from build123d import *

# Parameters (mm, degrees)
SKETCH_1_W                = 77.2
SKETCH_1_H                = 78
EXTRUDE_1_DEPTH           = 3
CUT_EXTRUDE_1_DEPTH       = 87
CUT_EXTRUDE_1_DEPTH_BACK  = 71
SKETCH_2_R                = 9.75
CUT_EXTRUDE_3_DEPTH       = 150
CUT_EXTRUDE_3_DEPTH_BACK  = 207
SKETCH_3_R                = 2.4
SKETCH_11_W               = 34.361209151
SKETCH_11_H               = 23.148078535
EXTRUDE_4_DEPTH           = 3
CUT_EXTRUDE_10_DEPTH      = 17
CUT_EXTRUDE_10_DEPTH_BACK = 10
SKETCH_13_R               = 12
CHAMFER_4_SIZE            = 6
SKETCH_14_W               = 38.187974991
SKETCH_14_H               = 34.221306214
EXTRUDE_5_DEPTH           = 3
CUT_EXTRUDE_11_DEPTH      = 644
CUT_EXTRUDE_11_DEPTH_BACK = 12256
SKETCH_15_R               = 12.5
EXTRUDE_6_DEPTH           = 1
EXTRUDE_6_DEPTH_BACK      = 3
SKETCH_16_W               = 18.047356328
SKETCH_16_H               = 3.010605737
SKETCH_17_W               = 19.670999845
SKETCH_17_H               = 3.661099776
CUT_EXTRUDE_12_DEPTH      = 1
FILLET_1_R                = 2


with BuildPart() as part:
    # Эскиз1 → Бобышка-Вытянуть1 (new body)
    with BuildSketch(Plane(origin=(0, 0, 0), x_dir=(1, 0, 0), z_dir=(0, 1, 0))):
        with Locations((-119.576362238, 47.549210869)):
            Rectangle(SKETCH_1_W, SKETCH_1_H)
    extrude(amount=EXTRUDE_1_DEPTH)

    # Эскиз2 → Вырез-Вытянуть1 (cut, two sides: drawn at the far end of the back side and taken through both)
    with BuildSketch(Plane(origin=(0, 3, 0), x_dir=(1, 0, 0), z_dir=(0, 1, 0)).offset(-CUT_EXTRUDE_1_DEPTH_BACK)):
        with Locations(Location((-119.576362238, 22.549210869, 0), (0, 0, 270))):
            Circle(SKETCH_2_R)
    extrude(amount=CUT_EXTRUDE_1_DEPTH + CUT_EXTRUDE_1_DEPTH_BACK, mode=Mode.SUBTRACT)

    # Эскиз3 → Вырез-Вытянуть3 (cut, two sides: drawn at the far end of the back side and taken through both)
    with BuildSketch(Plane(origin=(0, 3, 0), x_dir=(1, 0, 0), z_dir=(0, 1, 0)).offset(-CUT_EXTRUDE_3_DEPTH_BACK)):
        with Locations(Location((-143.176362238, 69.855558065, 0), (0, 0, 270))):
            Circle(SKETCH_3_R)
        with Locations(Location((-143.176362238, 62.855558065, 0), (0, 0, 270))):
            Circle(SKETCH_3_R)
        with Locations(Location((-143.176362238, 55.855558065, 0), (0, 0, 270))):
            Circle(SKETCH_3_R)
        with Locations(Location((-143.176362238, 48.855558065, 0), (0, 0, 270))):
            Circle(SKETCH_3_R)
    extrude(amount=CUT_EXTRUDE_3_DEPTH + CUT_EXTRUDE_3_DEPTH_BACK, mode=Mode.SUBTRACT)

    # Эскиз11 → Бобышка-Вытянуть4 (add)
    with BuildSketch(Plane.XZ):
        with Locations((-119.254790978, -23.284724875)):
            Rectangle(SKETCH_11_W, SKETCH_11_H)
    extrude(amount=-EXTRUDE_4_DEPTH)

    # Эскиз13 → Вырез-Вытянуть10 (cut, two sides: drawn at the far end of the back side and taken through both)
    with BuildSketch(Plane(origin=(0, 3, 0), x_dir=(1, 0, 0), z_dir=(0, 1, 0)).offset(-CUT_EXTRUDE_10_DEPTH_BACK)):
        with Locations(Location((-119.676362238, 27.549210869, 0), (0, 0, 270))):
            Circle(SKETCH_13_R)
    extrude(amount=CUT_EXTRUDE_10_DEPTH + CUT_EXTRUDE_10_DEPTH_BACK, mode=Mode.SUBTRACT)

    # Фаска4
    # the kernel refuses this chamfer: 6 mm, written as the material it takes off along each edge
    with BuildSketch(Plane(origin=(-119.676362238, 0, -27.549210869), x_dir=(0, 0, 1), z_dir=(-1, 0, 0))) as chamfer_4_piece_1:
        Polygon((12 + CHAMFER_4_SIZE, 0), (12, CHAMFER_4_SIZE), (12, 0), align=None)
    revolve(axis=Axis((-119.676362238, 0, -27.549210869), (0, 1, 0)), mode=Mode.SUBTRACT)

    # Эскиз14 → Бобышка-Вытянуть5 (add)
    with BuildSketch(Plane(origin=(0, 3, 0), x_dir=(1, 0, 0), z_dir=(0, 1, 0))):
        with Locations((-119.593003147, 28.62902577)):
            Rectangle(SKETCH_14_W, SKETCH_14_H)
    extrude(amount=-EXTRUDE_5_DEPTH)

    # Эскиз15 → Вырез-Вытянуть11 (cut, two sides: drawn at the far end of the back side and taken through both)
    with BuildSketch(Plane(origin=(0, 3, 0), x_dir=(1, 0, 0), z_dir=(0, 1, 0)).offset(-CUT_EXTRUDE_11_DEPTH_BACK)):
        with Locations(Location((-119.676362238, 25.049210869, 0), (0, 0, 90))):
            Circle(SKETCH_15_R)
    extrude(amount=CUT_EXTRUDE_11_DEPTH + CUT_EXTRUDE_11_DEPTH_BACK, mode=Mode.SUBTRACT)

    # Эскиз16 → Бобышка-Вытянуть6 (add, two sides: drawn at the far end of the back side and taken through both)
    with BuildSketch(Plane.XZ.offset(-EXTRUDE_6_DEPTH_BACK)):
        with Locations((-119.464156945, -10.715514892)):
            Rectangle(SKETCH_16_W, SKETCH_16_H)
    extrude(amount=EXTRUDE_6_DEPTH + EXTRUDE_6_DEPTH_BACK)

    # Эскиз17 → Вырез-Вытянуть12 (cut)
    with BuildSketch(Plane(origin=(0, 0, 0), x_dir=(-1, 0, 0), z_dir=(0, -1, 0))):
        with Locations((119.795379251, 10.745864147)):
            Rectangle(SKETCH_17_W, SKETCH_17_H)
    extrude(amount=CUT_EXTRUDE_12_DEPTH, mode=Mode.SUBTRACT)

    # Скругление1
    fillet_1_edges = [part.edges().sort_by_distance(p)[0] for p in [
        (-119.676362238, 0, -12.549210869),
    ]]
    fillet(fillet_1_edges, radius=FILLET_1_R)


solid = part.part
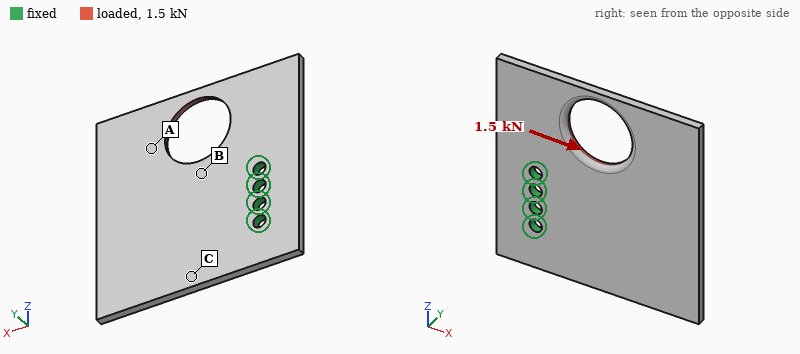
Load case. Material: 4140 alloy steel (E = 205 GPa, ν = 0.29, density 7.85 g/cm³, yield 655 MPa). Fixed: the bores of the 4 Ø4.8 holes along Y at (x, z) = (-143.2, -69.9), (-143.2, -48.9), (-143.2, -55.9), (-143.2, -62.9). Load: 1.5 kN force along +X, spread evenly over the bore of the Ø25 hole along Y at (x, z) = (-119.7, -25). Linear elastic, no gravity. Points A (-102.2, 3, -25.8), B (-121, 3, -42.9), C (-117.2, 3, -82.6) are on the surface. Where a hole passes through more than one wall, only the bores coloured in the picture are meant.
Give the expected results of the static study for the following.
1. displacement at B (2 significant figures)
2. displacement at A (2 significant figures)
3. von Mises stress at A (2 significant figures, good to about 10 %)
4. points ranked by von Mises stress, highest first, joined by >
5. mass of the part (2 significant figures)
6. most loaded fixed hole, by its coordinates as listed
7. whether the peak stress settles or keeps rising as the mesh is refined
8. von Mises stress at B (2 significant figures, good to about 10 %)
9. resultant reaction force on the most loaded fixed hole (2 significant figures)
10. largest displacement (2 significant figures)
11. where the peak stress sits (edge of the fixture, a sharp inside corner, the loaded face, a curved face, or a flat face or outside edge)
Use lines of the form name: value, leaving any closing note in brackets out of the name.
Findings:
displacement at B: 0.016 mm
displacement at A: 0.052 mm
von Mises stress at A: 21 MPa
points ranked by von Mises stress, highest first, joined by >: B > A > C
mass of the part: 130 g
most loaded fixed hole, by its coordinates as listed: (-143.2, -48.9)
whether the peak stress settles or keeps rising as the mesh is refined: keeps rising
von Mises stress at B: 37 MPa
resultant reaction force on the most loaded fixed hole: 2.5 kN
largest displacement: 0.10 mm
where the peak stress sits: edge of the fixture
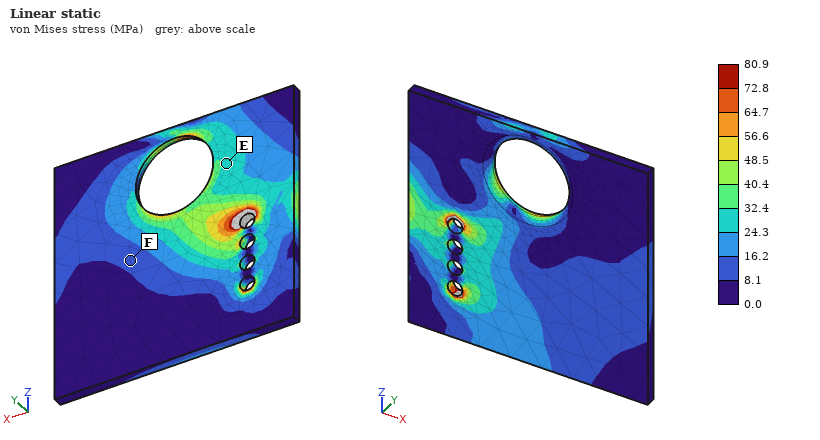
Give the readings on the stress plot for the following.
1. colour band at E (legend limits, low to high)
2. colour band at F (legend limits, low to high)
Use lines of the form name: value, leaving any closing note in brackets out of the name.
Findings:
colour band at E: 24.3 to 32.4 MPa
colour band at F: 8.1 to 16.2 MPa
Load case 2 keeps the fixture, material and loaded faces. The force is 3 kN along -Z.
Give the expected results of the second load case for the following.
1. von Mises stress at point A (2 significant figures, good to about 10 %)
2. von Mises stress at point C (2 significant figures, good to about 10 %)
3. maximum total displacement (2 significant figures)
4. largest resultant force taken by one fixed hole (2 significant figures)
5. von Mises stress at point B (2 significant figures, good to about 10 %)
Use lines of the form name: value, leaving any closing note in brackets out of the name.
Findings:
von Mises stress at point A: 41 MPa
von Mises stress at point C: 17 MPa
maximum total displacement: 0.12 mm
largest resultant force taken by one fixed hole: 3.0 kN
von Mises stress at point B: 50 MPa
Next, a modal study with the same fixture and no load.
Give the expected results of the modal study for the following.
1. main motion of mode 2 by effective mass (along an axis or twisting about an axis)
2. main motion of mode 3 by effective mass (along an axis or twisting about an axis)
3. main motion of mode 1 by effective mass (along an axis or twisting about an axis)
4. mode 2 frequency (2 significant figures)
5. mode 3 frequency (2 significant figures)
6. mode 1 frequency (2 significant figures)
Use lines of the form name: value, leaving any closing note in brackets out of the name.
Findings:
main motion of mode 2 by effective mass: twisting about X
main motion of mode 3 by effective mass: along Y
main motion of mode 1 by effective mass: along Y
mode 2 frequency: 1000 Hz
mode 3 frequency: 1800 Hz
mode 1 frequency: 560 Hz
